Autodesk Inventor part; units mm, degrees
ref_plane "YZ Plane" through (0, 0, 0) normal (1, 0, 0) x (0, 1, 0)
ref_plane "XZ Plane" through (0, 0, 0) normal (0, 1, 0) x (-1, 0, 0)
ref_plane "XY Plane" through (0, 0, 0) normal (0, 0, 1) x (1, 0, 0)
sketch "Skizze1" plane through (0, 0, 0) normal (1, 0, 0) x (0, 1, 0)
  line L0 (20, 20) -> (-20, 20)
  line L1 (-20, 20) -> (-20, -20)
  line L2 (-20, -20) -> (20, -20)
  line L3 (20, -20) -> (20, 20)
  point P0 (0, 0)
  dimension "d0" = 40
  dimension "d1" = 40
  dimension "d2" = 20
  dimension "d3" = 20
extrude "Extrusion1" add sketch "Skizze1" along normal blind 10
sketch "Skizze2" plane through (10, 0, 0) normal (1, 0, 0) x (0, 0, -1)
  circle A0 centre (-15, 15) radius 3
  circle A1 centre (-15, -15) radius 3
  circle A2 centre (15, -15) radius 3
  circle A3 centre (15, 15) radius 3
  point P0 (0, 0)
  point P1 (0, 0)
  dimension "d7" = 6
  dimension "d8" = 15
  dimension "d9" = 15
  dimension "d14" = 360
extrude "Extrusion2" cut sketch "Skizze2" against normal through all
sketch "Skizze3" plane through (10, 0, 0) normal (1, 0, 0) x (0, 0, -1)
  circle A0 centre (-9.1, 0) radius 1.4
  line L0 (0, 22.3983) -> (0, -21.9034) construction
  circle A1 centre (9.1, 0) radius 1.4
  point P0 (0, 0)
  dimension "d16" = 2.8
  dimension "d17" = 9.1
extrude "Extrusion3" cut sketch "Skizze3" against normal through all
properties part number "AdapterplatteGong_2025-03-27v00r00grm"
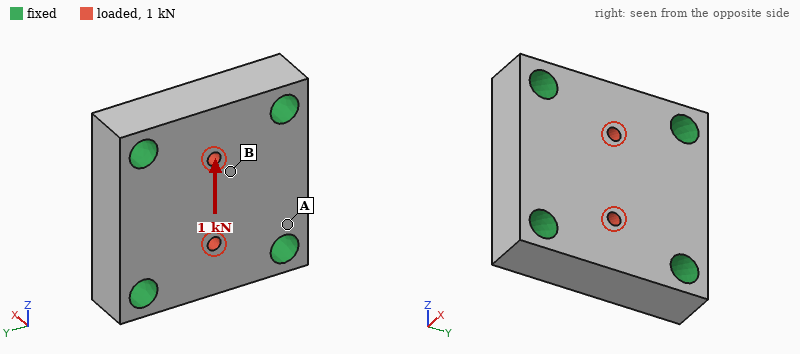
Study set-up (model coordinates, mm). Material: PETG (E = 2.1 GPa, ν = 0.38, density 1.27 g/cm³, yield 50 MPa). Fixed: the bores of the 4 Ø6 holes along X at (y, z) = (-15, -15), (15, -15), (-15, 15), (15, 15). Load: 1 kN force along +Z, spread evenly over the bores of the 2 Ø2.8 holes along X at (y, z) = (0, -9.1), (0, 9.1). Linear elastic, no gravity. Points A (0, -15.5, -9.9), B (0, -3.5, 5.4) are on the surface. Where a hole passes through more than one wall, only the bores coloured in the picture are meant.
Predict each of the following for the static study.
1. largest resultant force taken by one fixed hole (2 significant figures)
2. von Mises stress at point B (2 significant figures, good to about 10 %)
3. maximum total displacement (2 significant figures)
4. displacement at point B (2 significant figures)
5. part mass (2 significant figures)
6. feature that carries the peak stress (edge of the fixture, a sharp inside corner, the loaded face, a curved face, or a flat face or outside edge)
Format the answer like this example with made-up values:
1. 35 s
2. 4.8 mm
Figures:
1. 280 N
2. 3.0 MPa
3. 32 µm
4. 21 µm
5. 19 g
6. the loaded face
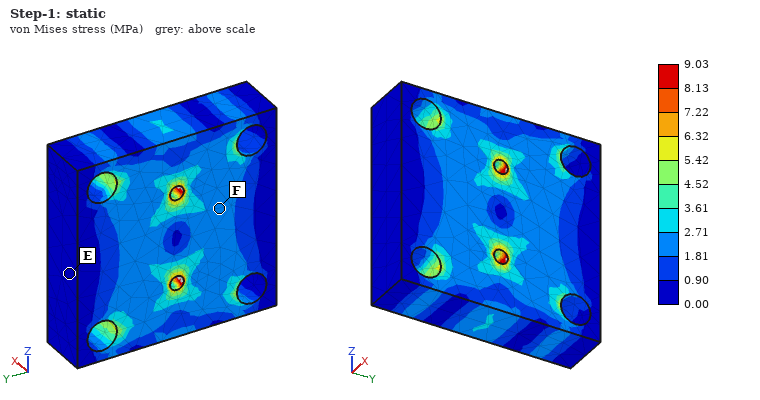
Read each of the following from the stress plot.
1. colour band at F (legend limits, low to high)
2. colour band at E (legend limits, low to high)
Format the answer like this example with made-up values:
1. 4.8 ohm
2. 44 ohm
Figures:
1. 1.81 to 2.71 MPa
2. 0.00 to 0.90 MPa
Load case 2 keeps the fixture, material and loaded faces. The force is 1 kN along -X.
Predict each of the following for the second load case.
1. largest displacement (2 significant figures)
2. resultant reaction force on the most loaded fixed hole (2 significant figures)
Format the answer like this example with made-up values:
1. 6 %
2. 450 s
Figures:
1. 73 µm
2. 250 N
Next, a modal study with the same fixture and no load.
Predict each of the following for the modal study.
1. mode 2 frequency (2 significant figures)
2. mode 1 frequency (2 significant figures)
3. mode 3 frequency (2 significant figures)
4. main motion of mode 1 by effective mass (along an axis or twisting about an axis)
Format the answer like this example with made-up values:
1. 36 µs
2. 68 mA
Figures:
1. 12 kHz
2. 8200 Hz
3. 12 kHz
4. along X
